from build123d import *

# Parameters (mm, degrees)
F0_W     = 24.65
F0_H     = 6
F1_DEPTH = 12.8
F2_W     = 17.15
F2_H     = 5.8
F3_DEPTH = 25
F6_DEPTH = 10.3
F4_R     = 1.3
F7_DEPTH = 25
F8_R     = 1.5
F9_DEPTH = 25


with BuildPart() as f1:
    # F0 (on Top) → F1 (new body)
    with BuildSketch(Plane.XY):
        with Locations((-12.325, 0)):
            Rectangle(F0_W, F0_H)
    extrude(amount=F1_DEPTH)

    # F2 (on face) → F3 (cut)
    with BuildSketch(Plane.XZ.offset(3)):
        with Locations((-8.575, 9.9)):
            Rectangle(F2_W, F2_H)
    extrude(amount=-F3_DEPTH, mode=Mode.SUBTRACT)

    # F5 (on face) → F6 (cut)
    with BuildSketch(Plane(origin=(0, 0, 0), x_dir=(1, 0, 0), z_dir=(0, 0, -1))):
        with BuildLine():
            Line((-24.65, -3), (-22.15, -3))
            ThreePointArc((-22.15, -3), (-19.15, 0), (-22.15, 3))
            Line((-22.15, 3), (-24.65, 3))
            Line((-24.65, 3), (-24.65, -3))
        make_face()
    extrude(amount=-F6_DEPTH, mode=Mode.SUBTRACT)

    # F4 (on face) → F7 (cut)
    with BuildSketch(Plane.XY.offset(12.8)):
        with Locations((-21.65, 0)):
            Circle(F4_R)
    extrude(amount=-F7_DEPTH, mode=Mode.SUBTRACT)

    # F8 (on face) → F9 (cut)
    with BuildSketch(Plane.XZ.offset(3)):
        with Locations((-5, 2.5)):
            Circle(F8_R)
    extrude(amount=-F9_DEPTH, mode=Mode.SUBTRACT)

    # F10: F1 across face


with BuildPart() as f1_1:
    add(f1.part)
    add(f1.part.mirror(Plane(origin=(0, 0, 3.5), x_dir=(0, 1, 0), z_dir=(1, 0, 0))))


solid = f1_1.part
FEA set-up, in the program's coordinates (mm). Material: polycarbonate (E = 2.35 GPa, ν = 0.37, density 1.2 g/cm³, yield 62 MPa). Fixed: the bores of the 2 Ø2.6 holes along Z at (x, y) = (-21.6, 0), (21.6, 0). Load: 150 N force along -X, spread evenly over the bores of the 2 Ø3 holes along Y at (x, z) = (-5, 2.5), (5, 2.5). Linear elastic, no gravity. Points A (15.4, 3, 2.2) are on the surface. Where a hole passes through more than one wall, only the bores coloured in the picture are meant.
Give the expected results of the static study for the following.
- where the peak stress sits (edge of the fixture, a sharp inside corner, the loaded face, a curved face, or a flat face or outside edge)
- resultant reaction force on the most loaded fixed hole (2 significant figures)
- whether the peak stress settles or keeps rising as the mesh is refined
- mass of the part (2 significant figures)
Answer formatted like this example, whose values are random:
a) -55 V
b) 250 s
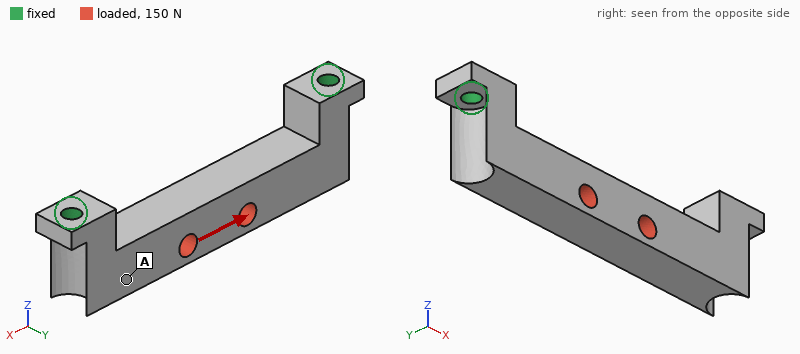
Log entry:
a) a sharp inside corner
b) 79 N
c) keeps rising
d) 2.3 g
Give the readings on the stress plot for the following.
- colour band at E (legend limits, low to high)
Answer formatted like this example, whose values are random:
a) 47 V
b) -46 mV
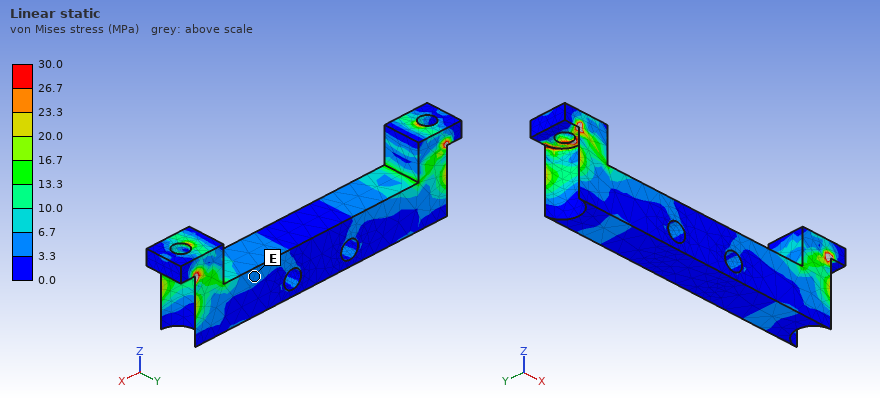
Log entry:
a) 3.3 to 6.7 MPa
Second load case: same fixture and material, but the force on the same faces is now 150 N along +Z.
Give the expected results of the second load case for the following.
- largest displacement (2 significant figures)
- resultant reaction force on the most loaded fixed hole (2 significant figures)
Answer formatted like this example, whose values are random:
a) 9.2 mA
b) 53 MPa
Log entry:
a) 0.27 mm
b) 100 N
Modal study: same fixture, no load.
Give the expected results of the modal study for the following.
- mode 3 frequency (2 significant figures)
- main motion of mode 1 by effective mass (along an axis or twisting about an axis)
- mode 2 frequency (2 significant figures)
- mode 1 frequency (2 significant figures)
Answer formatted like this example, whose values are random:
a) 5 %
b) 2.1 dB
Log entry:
a) 3900 Hz
b) along Y
c) 3800 Hz
d) 1900 Hz
